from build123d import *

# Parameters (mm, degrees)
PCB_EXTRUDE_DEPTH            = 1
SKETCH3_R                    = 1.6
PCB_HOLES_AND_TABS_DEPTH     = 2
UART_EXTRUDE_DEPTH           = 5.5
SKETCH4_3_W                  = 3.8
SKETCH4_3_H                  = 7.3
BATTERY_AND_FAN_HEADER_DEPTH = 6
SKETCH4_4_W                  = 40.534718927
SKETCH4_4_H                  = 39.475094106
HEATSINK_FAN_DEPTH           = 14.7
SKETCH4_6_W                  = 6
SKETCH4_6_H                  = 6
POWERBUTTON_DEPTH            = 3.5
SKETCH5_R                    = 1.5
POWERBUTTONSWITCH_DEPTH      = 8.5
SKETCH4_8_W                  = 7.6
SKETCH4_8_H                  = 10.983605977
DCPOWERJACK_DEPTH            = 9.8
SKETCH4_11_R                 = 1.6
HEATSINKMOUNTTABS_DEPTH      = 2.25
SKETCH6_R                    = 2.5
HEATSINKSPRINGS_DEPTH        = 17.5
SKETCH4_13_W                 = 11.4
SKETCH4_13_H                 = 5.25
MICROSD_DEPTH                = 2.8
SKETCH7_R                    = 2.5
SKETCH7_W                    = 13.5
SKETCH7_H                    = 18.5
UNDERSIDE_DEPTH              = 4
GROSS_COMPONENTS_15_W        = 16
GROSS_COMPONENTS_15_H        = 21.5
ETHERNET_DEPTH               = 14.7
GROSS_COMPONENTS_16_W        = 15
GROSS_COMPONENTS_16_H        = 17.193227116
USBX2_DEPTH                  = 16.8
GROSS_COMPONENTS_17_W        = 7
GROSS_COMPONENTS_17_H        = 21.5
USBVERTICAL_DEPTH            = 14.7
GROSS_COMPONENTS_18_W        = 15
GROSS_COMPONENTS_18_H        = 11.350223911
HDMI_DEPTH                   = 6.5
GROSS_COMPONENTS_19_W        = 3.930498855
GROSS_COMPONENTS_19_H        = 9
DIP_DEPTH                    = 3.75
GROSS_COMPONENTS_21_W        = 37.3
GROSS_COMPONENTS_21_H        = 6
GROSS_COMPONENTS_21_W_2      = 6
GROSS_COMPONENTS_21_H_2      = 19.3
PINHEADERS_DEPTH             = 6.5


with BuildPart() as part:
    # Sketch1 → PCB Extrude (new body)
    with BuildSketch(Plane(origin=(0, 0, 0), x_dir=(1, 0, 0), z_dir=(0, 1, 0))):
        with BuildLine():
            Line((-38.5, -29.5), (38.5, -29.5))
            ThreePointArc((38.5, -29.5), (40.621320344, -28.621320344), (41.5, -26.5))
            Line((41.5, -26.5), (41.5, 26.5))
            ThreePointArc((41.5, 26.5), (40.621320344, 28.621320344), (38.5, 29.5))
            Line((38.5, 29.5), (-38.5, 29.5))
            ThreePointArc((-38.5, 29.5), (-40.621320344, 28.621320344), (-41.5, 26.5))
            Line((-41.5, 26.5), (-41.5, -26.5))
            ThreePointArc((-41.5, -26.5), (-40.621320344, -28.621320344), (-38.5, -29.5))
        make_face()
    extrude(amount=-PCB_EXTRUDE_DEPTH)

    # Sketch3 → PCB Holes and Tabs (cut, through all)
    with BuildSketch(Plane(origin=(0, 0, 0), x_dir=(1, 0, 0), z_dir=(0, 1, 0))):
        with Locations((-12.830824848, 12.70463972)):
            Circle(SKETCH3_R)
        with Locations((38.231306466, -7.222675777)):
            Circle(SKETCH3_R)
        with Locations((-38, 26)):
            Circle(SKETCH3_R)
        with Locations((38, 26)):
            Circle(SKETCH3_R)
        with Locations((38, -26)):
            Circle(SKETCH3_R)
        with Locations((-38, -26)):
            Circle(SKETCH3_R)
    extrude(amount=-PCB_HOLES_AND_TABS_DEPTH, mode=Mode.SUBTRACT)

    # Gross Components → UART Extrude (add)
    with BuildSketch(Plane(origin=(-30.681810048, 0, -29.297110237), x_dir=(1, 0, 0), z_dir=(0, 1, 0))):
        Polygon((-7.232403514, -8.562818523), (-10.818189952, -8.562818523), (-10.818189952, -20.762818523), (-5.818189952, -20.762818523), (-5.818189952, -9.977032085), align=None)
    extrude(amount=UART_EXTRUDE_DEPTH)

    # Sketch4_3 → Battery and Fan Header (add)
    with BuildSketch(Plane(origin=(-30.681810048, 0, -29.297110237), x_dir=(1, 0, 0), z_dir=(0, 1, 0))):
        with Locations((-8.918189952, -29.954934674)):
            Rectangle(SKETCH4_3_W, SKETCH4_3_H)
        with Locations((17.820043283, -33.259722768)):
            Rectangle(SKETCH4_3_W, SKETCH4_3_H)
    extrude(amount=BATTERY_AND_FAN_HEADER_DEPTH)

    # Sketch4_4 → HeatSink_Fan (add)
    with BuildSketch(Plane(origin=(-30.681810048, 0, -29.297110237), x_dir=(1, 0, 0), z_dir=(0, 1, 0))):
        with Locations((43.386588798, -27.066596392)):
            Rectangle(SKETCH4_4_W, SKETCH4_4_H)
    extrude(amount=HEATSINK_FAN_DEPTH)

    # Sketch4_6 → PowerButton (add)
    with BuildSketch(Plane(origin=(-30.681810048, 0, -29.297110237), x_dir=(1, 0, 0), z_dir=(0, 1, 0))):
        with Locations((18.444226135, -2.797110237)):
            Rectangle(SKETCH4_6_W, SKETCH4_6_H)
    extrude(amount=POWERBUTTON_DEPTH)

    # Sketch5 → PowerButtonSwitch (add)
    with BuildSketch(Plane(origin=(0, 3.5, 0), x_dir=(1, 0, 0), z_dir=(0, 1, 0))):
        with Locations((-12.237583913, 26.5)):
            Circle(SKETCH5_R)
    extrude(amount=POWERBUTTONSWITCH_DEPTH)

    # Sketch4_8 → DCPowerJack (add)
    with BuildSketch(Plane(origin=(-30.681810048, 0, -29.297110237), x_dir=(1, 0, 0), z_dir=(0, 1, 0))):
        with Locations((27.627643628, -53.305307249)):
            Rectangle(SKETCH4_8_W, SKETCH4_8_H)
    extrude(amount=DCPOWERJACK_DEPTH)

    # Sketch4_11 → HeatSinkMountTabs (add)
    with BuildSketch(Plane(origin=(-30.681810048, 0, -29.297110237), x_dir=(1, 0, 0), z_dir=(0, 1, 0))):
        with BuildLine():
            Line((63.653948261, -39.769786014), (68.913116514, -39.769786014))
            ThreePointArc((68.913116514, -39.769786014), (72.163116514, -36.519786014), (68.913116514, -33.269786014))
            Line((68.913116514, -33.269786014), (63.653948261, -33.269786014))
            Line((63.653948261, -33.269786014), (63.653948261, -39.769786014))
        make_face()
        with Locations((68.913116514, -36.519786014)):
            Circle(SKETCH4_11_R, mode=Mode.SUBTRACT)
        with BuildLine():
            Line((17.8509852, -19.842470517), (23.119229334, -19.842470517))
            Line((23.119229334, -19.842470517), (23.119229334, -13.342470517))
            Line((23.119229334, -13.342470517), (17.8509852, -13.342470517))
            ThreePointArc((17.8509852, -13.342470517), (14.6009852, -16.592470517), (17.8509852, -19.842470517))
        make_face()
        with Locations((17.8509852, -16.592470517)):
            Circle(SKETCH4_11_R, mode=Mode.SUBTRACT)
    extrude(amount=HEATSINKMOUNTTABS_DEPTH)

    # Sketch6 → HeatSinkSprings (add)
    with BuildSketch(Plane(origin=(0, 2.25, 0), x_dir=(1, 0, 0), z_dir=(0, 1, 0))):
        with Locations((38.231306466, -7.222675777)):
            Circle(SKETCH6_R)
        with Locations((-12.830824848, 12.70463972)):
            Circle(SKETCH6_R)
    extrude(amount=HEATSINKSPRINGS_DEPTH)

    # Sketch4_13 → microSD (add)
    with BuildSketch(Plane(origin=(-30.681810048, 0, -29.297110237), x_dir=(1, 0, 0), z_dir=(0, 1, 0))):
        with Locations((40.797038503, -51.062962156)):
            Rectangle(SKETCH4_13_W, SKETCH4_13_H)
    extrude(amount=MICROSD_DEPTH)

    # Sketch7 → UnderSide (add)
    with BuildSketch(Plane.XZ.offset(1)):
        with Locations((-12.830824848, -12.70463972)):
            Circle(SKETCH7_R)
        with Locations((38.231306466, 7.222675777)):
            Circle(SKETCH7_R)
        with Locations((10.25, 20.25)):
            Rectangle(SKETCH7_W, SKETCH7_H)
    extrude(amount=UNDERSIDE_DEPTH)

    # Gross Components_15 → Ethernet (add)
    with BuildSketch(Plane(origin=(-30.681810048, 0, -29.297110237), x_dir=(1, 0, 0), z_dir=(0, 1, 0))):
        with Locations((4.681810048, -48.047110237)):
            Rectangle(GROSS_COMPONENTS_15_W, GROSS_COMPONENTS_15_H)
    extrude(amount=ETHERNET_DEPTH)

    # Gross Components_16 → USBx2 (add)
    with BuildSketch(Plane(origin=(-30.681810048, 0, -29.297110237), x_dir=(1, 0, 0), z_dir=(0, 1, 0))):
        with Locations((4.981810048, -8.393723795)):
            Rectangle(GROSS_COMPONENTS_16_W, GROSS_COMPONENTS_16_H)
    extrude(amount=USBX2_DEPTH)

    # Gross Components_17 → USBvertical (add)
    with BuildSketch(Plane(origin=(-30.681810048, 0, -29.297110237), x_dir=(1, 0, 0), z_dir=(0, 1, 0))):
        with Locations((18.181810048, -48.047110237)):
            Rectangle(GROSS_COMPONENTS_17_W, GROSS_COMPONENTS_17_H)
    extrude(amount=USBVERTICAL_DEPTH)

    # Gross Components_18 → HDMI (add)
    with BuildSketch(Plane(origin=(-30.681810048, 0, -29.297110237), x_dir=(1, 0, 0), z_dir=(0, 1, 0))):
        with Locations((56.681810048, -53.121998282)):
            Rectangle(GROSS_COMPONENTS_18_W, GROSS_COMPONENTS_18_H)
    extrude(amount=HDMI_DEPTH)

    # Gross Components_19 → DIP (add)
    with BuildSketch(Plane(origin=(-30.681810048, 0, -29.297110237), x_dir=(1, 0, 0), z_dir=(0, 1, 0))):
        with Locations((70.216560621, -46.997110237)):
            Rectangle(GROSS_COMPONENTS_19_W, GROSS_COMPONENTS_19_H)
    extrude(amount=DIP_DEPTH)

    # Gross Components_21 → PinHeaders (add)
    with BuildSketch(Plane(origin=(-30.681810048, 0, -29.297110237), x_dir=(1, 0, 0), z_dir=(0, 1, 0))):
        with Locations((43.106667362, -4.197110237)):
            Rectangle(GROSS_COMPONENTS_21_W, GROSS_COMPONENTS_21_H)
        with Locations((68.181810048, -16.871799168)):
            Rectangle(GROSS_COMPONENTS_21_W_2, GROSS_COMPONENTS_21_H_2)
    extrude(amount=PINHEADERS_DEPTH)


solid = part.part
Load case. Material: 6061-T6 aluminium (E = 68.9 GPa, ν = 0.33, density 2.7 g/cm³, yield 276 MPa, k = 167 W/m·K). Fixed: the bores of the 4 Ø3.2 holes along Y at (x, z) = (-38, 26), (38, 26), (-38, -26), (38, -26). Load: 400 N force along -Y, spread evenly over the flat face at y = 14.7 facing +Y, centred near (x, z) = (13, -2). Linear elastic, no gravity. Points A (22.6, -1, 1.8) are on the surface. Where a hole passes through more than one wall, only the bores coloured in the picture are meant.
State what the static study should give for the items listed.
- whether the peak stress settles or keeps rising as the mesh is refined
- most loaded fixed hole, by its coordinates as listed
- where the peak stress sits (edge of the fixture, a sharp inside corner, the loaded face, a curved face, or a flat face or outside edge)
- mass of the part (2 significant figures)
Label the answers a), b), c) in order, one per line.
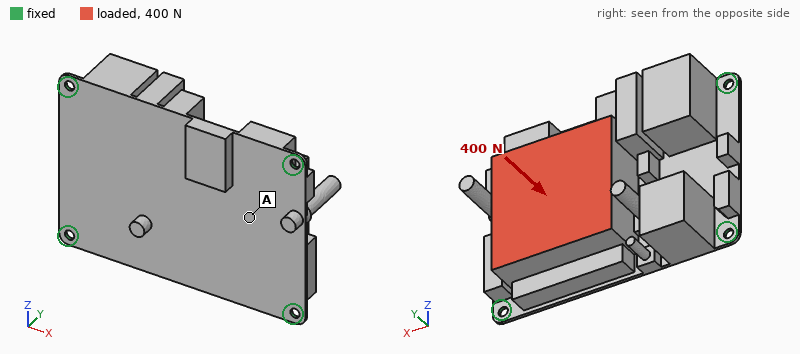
a) keeps rising
b) (38, -26)
c) edge of the fixture
d) 130 g
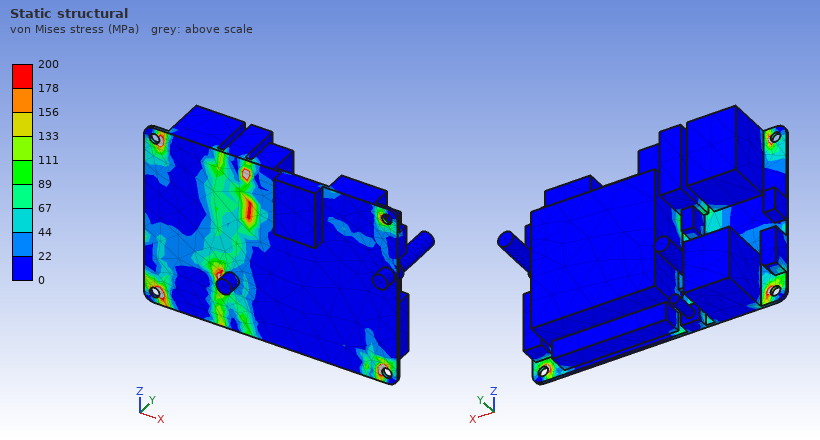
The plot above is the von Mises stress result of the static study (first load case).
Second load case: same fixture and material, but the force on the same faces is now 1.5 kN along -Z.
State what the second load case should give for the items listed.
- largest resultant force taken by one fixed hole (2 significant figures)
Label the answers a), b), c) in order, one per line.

a) 840 N
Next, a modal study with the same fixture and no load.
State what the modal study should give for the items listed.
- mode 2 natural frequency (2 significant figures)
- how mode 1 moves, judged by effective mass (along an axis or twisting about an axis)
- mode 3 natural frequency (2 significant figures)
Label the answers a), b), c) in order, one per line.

a) 1800 Hz
b) along Y
c) 2000 Hz
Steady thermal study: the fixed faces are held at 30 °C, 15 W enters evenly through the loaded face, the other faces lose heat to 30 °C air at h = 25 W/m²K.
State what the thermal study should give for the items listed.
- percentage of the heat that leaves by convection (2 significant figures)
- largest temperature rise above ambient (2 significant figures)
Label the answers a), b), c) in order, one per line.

a) 26 %
b) 13 K
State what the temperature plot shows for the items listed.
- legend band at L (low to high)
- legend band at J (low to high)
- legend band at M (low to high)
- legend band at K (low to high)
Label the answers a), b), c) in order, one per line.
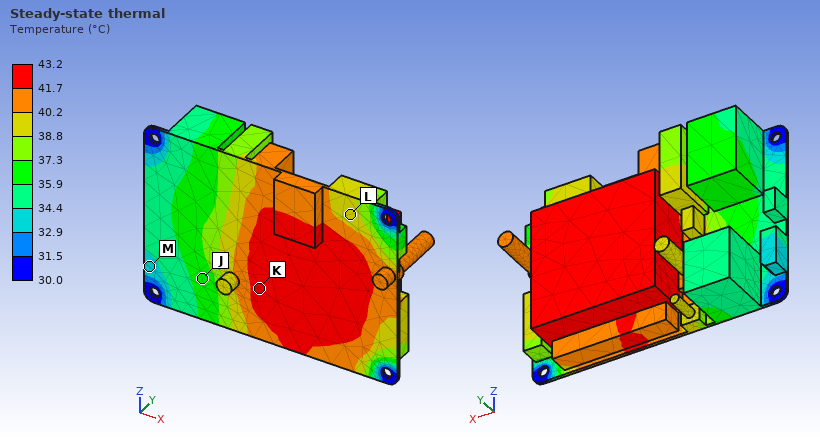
a) 38.8 to 40.2 °C
b) 35.9 to 37.3 °C
c) 32.9 to 34.4 °C
d) 41.7 to 43.2 °C
